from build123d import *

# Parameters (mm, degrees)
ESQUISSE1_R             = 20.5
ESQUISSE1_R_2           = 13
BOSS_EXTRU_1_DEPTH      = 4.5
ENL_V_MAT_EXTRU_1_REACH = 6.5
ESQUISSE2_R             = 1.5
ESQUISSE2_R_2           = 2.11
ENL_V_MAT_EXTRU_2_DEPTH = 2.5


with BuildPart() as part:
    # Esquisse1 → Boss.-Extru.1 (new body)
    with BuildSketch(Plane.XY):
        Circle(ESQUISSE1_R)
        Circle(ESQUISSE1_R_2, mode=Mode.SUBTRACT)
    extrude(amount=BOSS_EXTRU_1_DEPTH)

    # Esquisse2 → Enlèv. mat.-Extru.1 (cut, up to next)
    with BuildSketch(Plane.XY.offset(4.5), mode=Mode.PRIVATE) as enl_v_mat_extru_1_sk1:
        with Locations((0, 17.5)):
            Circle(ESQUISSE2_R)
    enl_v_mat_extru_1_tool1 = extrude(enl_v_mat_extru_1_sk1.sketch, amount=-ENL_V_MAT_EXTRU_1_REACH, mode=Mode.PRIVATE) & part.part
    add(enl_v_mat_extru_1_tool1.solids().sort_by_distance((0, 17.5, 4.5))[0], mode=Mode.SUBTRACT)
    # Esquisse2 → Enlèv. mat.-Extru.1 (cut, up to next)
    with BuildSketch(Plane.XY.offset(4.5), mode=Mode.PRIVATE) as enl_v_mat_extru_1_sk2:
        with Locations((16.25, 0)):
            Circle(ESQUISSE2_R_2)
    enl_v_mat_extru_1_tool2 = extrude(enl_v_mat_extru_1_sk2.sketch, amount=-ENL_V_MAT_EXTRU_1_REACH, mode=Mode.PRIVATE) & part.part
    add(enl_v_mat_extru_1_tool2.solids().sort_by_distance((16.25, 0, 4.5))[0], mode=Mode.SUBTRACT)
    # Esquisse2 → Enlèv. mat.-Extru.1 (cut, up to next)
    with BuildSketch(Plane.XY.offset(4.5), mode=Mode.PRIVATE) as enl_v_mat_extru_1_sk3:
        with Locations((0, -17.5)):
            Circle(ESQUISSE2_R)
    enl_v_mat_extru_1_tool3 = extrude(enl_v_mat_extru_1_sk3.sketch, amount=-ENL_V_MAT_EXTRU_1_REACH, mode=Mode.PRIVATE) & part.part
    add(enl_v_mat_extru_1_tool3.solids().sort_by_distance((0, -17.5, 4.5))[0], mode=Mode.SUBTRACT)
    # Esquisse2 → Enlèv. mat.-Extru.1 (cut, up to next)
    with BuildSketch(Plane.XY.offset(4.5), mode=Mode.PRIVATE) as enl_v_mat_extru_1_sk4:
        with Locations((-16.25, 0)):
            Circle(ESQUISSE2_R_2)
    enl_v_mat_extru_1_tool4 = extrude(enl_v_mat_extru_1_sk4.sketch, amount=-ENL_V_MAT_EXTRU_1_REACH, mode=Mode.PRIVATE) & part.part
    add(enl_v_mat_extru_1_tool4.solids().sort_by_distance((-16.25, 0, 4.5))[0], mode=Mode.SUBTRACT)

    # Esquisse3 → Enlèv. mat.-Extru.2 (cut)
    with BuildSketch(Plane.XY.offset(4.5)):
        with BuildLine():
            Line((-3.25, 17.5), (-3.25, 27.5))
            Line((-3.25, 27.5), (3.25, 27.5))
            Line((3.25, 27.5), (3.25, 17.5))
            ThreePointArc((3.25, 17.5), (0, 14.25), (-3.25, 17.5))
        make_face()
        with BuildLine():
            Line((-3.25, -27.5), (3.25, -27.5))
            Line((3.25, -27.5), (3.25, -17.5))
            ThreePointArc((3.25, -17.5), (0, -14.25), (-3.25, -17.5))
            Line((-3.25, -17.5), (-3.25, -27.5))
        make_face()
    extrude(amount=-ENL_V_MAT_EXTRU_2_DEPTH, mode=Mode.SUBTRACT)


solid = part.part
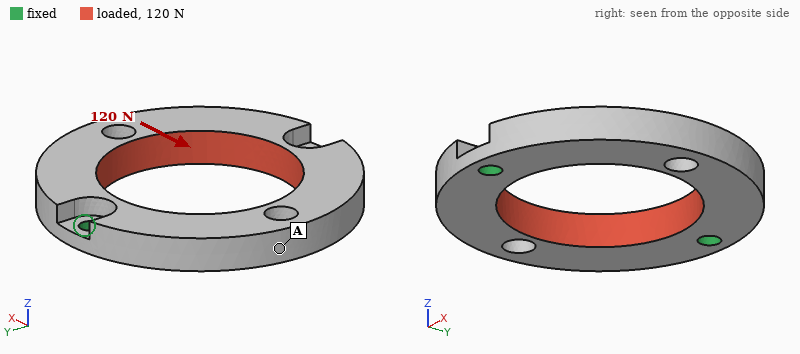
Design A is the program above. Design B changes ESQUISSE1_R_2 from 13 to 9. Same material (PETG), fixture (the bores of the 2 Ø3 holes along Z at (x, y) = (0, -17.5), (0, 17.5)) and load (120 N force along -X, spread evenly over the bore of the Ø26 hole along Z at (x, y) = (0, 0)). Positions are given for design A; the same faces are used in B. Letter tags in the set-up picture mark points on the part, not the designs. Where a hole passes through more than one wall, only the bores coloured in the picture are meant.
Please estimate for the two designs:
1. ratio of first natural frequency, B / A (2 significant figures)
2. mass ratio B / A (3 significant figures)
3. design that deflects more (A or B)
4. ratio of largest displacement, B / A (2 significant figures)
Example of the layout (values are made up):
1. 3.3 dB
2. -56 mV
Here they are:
1. 1.0
2. 1.39
3. A
4. 0.81
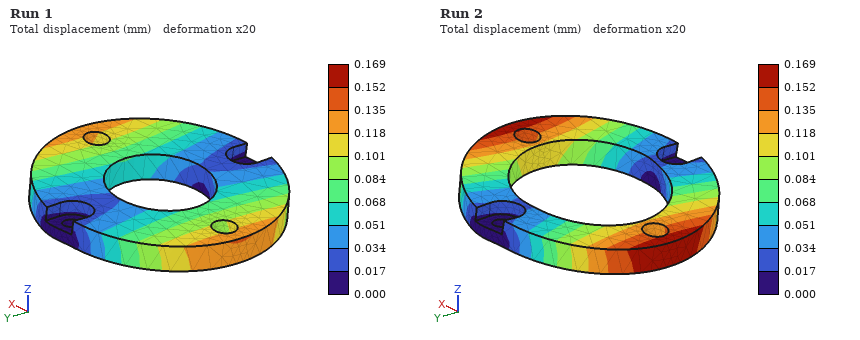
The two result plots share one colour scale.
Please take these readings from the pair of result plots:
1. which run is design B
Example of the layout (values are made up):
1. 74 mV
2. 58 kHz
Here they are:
1. Run 1
